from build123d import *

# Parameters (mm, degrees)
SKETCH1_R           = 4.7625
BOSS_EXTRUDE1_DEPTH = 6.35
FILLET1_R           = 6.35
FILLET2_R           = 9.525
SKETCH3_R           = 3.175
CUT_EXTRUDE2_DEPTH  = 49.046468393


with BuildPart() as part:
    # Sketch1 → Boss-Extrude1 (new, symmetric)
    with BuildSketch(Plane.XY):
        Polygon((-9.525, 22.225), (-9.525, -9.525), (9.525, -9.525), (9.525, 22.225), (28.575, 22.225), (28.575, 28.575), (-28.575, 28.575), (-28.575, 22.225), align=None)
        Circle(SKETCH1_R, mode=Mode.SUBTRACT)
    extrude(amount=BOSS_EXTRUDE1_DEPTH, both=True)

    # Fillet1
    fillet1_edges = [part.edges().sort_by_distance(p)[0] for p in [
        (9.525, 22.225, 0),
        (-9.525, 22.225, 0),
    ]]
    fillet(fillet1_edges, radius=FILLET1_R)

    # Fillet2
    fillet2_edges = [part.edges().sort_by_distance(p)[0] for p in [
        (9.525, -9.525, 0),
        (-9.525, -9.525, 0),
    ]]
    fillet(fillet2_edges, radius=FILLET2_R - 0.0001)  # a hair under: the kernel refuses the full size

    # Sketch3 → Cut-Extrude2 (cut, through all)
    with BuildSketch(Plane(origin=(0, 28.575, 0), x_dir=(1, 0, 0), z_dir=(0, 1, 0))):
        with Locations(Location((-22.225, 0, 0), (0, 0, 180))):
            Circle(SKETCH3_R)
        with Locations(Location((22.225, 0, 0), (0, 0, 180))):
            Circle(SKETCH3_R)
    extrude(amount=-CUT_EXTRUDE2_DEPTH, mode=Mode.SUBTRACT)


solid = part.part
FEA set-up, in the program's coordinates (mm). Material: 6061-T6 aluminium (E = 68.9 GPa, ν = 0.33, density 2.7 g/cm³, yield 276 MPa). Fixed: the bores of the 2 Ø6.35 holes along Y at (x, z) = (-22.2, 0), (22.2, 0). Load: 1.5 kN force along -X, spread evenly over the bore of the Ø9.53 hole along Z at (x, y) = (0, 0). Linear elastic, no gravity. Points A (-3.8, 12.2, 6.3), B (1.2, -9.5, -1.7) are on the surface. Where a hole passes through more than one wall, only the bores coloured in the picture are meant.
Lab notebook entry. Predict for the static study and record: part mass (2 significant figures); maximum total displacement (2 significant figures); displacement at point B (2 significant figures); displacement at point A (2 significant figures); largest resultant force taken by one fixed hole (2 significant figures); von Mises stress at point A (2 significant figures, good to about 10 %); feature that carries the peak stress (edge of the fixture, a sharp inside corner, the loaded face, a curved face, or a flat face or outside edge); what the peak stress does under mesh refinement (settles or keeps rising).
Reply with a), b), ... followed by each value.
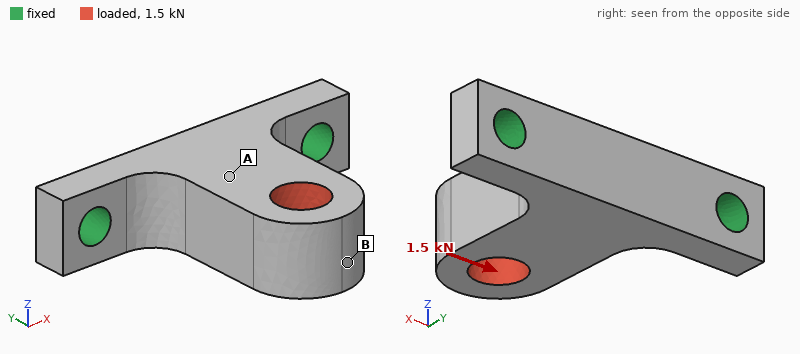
a) 29 g
b) 54 µm
c) 54 µm
d) 14 µm
e) 1.4 kN
f) 16 MPa
g) edge of the fixture
h) keeps rising
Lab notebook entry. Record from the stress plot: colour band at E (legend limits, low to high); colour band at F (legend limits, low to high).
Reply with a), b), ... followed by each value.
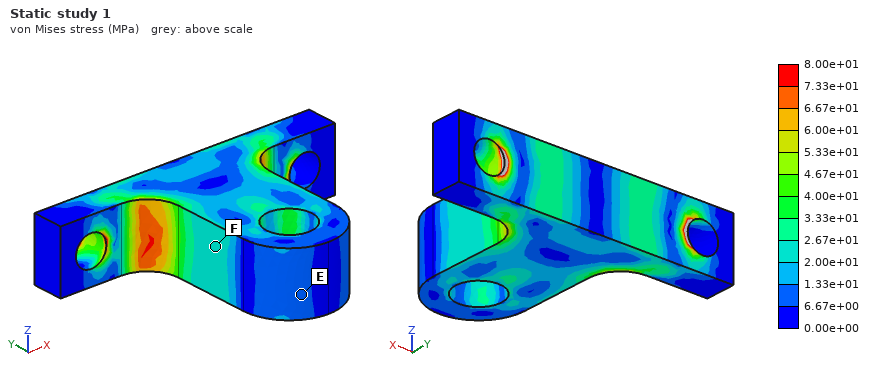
a) 6.67e+00 to 1.33e+01 MPa
b) 2.00e+01 to 2.67e+01 MPa
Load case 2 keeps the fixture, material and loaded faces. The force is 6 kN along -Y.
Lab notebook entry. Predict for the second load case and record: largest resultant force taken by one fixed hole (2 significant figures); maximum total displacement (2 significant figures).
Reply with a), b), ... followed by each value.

a) 3.5 kN
b) 52 µm
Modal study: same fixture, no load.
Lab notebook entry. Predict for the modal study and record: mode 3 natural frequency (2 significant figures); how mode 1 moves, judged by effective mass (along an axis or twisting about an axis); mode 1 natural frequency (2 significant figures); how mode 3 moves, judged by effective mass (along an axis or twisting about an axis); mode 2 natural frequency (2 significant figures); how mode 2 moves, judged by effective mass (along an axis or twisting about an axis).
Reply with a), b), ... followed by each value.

a) 13 kHz
b) along Z
c) 3900 Hz
d) along Y
e) 10 kHz
f) along X
